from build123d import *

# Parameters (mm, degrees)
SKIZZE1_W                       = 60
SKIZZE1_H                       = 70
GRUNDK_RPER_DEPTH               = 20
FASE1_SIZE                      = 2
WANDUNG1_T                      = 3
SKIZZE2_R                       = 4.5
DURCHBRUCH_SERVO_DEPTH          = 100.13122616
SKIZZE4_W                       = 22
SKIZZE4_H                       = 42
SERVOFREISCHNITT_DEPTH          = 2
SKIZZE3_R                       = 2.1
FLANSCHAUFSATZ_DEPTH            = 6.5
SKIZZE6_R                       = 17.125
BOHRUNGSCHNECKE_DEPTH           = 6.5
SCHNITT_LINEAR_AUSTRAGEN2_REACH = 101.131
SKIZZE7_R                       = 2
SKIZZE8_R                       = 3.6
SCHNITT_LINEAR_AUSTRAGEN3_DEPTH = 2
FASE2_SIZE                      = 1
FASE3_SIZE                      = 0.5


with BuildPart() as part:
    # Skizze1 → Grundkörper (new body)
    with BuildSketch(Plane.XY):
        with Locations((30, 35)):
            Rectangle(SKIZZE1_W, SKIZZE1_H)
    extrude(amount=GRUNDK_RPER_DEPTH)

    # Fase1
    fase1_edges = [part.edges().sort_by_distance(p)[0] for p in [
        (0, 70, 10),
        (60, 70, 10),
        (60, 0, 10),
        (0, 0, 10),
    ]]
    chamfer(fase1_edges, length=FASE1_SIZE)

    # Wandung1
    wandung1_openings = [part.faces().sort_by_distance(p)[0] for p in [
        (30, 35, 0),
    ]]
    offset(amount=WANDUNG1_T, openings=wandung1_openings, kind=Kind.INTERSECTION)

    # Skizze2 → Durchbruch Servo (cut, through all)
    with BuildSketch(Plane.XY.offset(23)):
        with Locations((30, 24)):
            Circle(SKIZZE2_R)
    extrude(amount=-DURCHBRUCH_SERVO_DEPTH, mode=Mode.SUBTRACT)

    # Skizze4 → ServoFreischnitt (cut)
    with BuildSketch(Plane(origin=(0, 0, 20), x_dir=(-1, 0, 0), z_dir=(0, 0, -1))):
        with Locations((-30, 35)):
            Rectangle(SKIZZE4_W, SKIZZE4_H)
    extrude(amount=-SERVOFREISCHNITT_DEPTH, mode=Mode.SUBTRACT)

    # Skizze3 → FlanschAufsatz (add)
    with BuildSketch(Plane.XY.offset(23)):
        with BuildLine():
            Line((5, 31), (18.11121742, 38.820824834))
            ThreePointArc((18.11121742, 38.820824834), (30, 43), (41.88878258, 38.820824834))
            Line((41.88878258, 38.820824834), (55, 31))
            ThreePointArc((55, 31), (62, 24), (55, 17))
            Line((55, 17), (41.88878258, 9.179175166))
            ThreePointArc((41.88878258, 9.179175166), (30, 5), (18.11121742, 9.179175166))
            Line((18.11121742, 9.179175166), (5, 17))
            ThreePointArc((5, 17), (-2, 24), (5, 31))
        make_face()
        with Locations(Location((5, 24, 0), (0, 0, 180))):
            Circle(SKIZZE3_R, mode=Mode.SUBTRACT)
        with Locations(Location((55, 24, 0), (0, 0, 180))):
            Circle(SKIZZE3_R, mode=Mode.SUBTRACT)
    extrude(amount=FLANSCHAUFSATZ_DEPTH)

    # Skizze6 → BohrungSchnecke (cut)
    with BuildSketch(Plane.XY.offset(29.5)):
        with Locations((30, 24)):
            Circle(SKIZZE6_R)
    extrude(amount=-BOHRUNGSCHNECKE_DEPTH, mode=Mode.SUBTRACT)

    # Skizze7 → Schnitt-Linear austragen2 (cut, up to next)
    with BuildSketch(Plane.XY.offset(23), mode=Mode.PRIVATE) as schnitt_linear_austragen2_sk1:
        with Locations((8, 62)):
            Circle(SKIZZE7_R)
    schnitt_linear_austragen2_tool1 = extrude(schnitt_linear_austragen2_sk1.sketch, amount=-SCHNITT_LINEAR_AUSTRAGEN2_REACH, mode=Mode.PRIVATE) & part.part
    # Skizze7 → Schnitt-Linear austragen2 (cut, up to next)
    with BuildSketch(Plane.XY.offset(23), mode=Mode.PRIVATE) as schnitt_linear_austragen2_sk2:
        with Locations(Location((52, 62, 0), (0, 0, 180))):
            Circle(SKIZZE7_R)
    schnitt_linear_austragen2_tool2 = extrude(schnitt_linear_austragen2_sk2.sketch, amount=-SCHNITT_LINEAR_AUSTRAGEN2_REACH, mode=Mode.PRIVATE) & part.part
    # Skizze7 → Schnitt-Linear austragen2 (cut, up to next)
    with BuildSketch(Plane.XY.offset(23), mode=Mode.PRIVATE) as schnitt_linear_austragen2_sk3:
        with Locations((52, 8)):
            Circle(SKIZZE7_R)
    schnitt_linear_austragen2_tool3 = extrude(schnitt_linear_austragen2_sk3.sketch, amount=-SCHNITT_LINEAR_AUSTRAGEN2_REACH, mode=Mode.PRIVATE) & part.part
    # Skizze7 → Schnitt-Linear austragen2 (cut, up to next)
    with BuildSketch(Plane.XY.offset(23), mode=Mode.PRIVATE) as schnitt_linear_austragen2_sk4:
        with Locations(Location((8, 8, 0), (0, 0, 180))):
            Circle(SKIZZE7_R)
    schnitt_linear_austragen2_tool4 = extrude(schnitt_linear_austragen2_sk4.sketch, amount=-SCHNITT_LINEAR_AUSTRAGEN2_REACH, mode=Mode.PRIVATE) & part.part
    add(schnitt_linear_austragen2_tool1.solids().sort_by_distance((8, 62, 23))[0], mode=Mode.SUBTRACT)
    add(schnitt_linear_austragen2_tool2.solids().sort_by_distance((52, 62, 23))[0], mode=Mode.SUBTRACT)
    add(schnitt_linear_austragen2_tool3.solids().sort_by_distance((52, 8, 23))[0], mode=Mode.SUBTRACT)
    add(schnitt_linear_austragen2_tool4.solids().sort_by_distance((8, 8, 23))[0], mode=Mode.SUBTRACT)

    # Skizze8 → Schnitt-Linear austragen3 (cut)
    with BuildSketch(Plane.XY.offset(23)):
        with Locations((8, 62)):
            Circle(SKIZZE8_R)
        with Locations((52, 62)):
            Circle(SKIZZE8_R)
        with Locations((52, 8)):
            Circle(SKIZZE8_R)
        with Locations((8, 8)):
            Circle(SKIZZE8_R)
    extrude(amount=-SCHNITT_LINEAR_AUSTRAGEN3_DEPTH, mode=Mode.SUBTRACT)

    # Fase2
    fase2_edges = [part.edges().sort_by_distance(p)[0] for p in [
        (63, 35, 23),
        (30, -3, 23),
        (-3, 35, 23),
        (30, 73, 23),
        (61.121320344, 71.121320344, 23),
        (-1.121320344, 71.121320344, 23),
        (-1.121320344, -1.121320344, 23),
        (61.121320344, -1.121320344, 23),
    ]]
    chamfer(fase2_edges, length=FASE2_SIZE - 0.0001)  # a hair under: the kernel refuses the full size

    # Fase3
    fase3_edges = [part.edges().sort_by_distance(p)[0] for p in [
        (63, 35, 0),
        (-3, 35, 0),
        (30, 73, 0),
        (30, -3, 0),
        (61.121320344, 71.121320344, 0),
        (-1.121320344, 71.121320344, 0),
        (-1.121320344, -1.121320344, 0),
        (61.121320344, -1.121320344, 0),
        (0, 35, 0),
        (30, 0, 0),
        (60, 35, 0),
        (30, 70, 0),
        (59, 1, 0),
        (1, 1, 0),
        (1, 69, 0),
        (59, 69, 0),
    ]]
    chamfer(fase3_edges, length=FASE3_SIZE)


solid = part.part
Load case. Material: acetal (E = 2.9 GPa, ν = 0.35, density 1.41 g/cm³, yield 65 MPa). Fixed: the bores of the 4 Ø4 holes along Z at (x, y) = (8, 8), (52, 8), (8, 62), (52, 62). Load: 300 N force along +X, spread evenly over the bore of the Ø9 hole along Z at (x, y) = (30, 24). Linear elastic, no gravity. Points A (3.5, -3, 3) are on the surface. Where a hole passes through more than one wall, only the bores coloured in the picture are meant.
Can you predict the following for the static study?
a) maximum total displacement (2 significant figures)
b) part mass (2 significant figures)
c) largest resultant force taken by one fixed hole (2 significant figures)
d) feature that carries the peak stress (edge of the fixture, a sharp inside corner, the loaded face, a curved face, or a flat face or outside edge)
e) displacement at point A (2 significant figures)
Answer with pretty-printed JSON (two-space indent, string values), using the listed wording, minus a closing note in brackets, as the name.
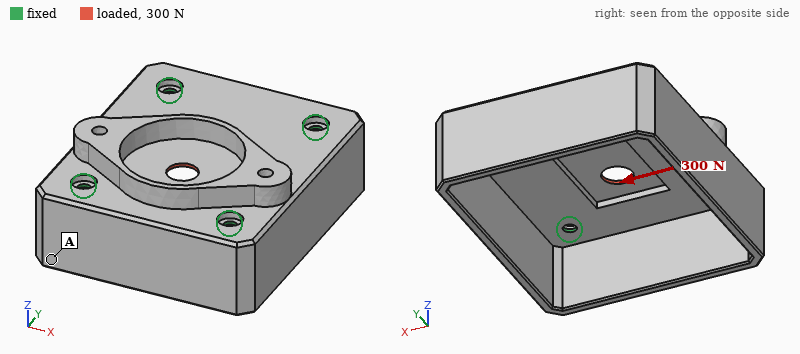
{
  "maximum total displacement": "58 µm",
  "part mass": "46 g",
  "largest resultant force taken by one fixed hole": "110 N",
  "feature that carries the peak stress": "the loaded face",
  "displacement at point A": "11 µm"
}
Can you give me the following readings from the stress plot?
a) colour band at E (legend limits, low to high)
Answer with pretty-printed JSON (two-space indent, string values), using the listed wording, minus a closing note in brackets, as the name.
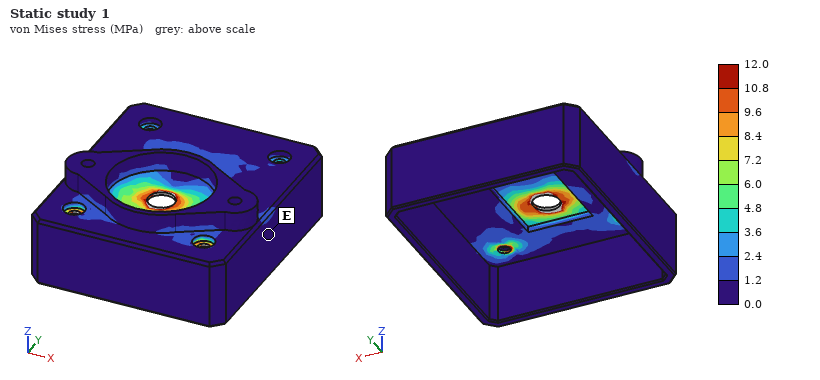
{
  "colour band at E": "0.0 to 1.2 MPa"
}
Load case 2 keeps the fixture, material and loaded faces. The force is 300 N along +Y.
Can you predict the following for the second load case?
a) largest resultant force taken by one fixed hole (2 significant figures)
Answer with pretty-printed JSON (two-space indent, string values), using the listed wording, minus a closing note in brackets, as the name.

{
  "largest resultant force taken by one fixed hole": "91 N"
}
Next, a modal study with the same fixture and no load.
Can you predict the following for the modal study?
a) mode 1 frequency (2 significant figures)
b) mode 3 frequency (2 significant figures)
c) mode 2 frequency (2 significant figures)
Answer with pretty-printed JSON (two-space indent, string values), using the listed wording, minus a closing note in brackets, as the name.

{
  "mode 1 frequency": "1400 Hz",
  "mode 3 frequency": "1400 Hz",
  "mode 2 frequency": "1400 Hz"
}
